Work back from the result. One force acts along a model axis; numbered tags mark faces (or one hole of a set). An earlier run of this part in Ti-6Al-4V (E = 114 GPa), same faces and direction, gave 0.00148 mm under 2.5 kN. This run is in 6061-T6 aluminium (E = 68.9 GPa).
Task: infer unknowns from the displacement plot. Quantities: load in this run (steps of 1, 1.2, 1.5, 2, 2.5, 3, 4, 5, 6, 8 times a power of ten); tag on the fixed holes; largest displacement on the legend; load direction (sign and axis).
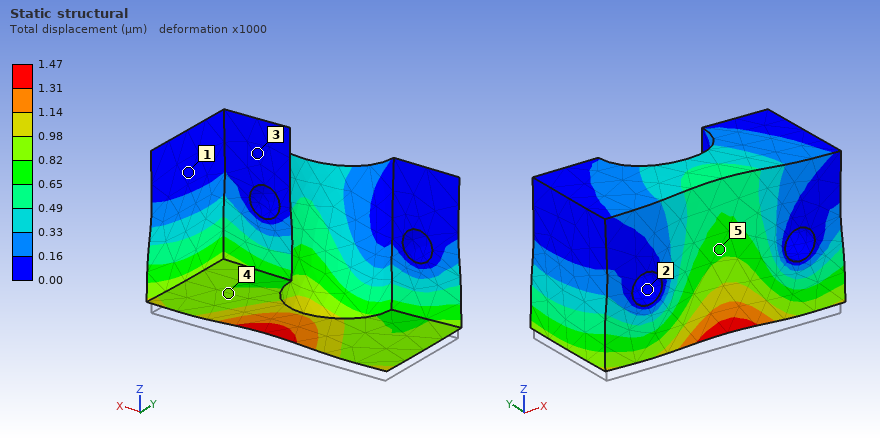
1.5 kN
2
1.47 µm
+Z
